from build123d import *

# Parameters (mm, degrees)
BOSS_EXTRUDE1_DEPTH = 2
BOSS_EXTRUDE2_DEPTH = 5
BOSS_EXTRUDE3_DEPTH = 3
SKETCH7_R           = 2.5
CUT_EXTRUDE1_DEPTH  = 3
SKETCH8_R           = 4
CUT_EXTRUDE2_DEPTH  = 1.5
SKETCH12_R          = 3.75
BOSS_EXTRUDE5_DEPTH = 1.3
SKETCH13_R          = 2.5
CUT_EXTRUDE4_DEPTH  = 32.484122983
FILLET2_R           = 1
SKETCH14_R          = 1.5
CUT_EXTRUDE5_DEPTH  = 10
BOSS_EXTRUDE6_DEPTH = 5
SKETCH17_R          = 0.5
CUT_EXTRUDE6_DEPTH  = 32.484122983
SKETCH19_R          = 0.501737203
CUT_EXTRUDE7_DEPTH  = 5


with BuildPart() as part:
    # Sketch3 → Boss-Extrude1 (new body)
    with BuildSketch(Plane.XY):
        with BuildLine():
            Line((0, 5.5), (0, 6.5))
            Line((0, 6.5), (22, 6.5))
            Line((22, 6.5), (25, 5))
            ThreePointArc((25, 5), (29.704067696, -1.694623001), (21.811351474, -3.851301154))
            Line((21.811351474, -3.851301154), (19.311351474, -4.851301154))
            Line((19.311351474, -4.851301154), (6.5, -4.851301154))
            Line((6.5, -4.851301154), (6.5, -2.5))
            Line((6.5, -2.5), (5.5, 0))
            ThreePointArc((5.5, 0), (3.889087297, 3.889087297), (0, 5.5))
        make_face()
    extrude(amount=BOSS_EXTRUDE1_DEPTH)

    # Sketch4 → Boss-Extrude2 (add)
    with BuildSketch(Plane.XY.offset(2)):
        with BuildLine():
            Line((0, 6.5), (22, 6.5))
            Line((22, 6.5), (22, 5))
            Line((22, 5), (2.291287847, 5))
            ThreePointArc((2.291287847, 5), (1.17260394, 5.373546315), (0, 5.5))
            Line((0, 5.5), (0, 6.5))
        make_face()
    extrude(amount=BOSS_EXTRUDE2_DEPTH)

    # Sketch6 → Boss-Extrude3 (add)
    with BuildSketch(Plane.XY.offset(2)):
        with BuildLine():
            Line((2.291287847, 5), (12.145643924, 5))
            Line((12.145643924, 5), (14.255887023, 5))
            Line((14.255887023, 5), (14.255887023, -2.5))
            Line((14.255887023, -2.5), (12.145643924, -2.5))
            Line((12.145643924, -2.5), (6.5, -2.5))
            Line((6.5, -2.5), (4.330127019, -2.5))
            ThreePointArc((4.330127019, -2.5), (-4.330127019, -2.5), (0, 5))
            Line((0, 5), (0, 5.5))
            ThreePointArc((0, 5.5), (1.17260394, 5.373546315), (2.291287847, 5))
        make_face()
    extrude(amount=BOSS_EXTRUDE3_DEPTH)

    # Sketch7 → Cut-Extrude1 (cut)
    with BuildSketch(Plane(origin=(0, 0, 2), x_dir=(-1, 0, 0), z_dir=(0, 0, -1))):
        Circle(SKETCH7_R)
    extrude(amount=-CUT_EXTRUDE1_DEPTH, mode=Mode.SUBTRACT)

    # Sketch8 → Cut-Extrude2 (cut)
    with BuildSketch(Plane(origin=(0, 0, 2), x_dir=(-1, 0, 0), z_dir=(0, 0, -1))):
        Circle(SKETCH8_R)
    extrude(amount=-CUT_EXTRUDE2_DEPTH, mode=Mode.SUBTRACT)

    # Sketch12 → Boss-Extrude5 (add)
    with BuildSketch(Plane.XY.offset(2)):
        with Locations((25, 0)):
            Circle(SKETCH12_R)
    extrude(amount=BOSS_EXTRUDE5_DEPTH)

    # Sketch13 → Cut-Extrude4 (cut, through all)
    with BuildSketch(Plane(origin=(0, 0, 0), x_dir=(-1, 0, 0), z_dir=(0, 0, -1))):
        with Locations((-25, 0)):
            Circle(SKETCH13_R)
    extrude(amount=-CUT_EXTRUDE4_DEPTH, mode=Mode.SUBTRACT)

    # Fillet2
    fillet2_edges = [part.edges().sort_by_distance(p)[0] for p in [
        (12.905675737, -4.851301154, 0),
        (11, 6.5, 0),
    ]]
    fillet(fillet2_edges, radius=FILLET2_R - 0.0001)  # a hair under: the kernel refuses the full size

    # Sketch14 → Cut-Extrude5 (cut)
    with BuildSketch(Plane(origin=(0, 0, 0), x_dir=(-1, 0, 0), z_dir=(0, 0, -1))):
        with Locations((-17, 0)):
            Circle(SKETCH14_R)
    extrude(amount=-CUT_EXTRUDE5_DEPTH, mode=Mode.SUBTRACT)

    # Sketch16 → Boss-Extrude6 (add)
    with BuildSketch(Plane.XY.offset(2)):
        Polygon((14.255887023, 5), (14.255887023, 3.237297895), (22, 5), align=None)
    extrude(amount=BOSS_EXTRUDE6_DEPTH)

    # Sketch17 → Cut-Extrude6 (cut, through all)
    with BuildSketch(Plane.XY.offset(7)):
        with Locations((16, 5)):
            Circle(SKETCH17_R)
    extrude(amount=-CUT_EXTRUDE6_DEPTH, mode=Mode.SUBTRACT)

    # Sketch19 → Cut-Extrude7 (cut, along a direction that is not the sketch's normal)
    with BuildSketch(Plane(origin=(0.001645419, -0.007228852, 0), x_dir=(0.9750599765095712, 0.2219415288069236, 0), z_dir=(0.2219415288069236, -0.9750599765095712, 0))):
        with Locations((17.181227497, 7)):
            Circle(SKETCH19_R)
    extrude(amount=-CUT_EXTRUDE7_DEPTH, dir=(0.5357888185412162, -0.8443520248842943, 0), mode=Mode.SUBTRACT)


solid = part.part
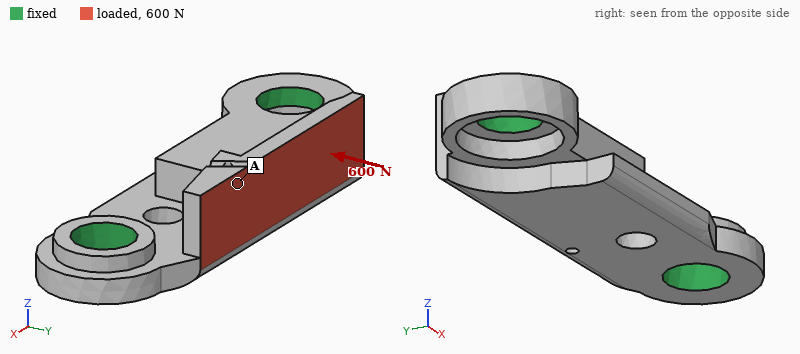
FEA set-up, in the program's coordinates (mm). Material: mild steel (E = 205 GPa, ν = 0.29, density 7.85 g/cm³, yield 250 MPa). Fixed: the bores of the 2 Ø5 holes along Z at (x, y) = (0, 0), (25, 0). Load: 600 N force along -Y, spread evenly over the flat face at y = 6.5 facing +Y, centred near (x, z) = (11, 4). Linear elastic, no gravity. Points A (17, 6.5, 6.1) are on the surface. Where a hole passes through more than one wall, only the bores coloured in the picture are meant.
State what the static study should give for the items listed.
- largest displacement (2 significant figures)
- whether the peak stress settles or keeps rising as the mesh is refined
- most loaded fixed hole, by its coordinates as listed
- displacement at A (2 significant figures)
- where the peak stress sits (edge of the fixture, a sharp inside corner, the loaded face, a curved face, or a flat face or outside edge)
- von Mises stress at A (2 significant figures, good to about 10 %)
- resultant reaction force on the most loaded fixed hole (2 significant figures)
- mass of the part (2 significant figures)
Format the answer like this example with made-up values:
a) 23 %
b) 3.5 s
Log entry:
a) 9.3 µm
b) keeps rising
c) (0, 0)
d) 7.5 µm
e) edge of the fixture
f) 14 MPa
g) 370 N
h) 8.2 g
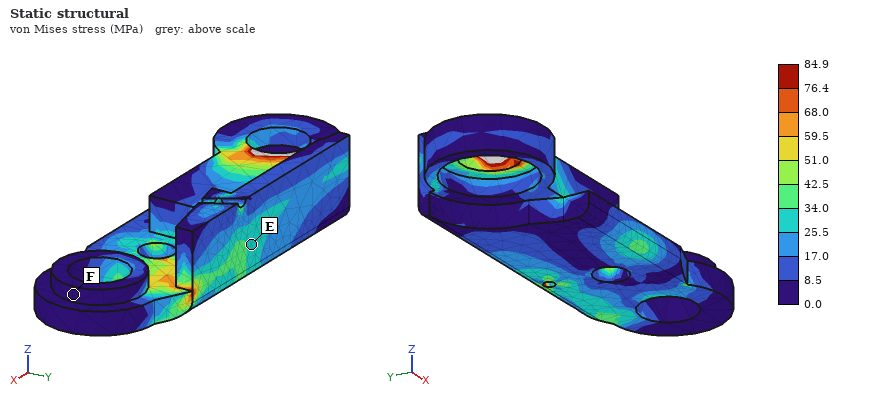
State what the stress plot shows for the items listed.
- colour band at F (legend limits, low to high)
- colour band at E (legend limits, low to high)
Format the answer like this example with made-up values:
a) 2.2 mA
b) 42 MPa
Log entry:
a) 0.0 to 8.5 MPa
b) 25.5 to 34.0 MPa
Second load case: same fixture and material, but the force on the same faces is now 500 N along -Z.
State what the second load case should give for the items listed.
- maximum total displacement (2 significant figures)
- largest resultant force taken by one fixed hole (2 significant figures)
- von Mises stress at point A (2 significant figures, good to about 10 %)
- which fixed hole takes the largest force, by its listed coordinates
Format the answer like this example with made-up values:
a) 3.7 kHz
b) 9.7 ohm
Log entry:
a) 16 µm
b) 280 N
c) 36 MPa
d) (0, 0)
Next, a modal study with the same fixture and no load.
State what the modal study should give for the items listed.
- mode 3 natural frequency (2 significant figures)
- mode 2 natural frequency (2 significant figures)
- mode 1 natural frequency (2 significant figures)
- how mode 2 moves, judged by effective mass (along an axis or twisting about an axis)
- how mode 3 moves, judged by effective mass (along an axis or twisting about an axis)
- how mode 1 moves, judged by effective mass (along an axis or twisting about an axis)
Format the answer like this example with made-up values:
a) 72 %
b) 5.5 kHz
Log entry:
a) 35 kHz
b) 25 kHz
c) 20 kHz
d) along Z
e) along Y
f) along Z
